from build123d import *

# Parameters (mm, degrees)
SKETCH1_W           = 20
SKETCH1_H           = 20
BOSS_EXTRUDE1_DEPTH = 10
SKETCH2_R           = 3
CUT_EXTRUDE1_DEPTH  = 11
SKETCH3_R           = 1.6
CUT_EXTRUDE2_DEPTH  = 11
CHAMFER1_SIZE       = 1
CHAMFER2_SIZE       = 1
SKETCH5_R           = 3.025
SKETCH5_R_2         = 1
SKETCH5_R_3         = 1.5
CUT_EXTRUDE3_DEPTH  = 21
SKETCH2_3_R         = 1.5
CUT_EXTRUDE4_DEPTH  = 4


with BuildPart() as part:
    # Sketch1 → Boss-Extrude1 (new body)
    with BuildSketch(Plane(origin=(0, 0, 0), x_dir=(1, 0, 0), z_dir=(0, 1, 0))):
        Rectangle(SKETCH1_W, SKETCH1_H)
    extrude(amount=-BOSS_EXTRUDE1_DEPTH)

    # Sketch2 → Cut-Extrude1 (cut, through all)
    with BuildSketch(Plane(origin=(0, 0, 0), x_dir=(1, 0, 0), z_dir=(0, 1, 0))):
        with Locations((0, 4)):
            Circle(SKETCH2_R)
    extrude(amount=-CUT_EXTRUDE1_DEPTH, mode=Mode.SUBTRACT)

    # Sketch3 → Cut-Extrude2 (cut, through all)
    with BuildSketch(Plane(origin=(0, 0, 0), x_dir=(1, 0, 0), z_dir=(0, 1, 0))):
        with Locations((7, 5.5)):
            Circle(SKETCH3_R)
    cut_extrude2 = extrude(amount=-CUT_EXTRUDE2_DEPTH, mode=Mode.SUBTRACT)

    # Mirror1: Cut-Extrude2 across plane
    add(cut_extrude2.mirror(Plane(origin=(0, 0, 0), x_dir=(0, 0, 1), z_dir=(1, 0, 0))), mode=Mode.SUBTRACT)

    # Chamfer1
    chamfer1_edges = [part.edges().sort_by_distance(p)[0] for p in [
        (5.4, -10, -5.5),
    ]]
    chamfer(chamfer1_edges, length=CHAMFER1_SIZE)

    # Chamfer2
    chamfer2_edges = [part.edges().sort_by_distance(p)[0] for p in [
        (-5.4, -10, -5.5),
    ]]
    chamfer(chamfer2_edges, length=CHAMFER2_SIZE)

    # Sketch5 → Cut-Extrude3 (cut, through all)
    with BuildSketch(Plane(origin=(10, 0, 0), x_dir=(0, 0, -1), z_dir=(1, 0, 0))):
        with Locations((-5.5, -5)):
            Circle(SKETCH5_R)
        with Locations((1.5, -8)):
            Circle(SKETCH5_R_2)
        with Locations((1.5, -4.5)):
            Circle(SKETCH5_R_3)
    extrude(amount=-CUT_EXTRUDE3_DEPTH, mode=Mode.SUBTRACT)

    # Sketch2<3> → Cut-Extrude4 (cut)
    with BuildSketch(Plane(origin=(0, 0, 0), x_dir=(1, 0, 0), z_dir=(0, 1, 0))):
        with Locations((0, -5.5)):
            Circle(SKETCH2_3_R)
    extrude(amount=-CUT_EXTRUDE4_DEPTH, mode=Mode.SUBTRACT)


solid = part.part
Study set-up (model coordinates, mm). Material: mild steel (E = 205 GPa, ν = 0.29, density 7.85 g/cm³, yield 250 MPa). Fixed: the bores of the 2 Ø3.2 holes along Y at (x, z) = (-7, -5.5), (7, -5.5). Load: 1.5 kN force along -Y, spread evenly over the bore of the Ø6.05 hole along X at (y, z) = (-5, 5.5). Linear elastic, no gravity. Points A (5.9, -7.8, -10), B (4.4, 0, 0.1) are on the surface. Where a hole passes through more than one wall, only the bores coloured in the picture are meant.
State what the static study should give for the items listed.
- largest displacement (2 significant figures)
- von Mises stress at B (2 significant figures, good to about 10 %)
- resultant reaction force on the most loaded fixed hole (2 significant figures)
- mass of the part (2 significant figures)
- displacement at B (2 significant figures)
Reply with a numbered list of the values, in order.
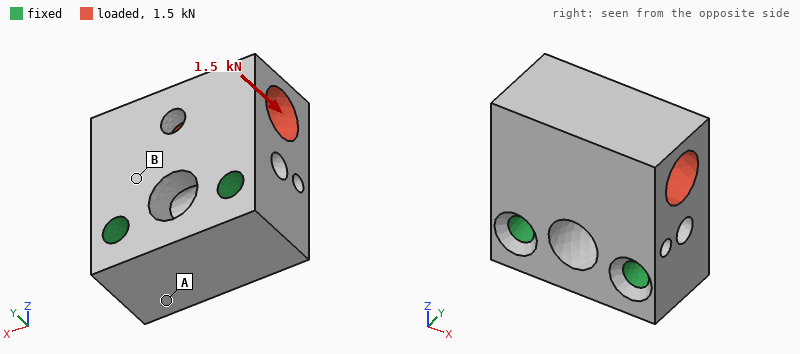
1. 11 µm
2. 28 MPa
3. 750 N
4. 22 g
5. 3.3 µm
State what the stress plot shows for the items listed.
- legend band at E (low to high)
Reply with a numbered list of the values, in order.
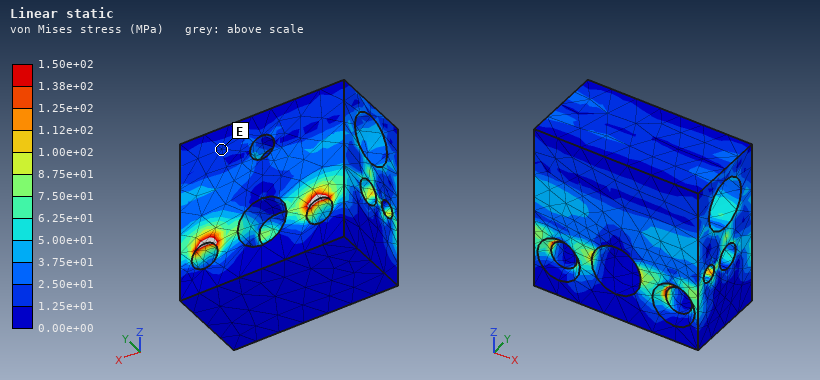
1. 1.25e+01 to 2.50e+01 MPa
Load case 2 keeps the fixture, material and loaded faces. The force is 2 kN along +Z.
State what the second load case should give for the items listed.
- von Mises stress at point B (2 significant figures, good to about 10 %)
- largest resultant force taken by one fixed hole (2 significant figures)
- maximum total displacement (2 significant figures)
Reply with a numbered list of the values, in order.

1. 19 MPa
2. 1.0 kN
3. 2.1 µm
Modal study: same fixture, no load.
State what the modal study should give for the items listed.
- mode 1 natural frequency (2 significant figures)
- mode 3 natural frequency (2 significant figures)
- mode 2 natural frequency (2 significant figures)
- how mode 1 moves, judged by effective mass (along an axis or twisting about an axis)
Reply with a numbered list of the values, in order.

1. 21 kHz
2. 36 kHz
3. 34 kHz
4. along Y
